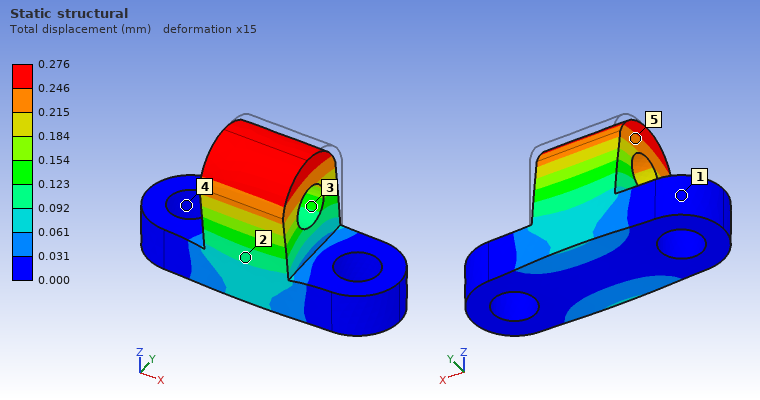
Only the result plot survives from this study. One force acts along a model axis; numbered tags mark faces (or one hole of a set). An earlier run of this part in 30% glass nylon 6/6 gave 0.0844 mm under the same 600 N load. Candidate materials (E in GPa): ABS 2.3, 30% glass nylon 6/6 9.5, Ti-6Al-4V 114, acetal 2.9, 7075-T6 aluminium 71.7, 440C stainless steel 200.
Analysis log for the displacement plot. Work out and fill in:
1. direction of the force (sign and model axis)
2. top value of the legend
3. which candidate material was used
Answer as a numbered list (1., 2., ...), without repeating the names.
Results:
1. -Y
2. 0.276 mm
3. acetal
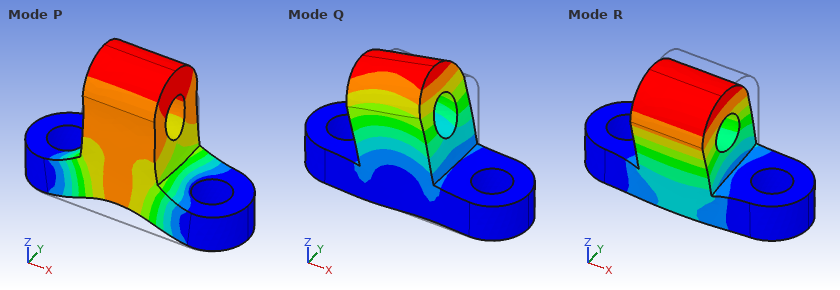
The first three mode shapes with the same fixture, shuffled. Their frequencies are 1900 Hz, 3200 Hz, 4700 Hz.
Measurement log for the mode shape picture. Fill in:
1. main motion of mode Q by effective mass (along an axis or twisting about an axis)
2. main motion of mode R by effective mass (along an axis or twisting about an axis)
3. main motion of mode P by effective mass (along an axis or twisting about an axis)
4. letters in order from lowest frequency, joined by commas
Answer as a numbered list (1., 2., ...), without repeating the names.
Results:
1. along X
2. along Y
3. along Z
4. R, Q, P
